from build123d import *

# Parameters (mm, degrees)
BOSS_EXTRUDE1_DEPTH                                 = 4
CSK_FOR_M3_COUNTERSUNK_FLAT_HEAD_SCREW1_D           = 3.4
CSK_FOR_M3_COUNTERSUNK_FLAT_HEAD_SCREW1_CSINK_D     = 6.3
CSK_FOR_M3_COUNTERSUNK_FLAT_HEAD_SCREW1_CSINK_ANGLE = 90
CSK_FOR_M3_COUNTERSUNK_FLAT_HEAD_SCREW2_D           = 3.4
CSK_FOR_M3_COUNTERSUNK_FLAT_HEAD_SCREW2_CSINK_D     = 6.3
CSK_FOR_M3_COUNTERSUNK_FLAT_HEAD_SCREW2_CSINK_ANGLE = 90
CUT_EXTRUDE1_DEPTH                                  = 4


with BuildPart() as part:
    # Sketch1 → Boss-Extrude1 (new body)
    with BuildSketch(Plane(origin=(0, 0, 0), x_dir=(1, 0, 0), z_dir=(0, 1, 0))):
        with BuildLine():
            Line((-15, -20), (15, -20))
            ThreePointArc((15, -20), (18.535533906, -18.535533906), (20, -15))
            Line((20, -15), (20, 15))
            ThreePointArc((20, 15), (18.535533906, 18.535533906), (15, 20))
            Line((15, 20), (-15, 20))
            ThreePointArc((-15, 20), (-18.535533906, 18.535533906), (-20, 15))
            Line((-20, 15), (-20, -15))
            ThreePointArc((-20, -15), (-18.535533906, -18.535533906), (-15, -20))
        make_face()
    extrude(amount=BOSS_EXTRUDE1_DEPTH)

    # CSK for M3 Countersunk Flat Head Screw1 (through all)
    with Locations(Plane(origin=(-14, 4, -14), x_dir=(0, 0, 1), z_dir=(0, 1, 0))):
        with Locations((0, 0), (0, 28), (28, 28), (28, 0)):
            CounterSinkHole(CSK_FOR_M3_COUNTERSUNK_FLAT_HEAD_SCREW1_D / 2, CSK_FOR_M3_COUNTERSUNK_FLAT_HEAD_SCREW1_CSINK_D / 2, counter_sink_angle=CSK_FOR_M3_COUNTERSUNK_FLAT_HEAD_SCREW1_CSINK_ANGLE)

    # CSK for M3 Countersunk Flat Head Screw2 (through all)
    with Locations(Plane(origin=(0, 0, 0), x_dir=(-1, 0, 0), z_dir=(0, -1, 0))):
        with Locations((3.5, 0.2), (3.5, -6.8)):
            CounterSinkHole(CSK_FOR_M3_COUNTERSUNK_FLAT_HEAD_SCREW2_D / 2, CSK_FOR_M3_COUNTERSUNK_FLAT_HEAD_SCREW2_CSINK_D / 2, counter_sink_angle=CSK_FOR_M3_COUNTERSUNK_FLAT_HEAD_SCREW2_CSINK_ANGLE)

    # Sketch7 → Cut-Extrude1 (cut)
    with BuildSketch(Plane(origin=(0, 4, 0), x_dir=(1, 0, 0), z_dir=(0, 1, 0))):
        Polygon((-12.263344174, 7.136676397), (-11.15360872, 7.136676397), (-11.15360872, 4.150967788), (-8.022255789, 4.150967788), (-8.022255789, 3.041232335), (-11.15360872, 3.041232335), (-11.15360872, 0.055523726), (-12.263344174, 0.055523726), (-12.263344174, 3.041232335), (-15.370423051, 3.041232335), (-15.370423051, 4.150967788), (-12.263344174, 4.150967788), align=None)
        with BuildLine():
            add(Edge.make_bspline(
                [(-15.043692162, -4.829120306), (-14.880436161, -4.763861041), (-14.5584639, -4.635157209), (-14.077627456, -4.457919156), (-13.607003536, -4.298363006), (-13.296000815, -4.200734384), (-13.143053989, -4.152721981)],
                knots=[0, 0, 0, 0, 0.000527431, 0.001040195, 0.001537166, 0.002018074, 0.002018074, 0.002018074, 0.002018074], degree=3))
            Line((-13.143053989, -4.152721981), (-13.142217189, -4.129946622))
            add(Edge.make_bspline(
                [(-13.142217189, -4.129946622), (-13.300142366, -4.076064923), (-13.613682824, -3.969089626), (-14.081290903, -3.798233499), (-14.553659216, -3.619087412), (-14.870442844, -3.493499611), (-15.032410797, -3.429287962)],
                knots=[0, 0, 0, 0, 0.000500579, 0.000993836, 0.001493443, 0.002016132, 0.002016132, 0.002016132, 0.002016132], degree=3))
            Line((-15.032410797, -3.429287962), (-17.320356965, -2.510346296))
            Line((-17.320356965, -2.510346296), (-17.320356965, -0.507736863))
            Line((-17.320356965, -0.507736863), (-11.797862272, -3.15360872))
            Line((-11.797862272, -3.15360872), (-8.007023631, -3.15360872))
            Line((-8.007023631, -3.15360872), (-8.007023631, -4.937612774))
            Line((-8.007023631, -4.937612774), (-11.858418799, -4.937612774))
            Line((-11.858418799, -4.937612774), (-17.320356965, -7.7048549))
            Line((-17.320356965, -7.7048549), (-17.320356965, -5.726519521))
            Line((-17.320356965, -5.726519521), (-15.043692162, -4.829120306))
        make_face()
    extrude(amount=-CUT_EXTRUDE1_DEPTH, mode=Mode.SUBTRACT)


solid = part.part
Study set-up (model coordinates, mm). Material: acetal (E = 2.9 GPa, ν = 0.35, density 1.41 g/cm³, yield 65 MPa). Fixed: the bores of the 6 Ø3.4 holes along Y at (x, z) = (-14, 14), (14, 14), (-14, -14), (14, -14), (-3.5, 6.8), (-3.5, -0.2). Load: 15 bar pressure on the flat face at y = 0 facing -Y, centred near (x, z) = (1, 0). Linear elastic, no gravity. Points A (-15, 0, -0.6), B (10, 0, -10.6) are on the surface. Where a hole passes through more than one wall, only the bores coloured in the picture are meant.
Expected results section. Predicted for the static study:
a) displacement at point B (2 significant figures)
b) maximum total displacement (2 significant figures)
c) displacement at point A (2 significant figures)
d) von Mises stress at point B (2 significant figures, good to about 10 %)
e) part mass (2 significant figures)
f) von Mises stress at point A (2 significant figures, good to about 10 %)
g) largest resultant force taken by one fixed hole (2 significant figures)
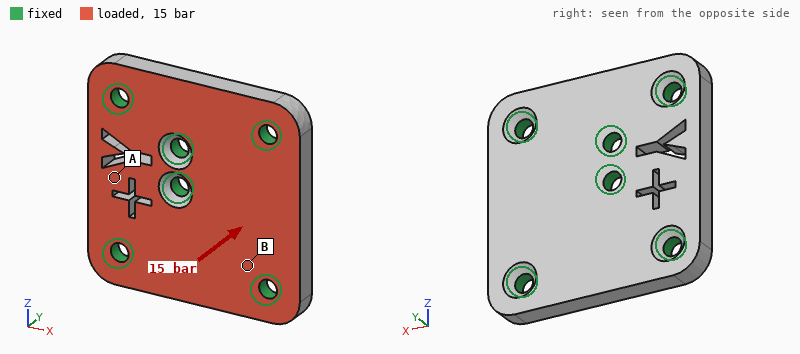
0.088 mm
0.23 mm
0.14 mm
17 MPa
8.2 g
8.0 MPa
470 N
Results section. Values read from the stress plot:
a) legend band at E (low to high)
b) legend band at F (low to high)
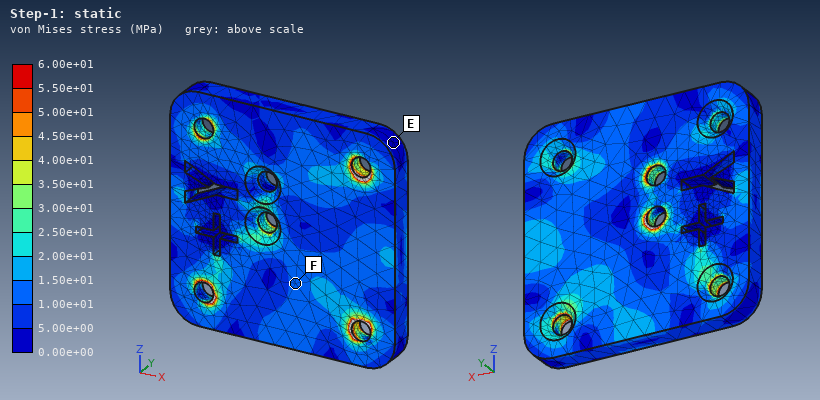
0.00e+00 to 5.00e+00 MPa
1.00e+01 to 1.50e+01 MPa
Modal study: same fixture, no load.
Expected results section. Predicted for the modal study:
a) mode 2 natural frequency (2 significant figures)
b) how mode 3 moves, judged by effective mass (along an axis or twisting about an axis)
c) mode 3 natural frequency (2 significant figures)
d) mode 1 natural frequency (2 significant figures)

6500 Hz
along Y
7000 Hz
6300 Hz
